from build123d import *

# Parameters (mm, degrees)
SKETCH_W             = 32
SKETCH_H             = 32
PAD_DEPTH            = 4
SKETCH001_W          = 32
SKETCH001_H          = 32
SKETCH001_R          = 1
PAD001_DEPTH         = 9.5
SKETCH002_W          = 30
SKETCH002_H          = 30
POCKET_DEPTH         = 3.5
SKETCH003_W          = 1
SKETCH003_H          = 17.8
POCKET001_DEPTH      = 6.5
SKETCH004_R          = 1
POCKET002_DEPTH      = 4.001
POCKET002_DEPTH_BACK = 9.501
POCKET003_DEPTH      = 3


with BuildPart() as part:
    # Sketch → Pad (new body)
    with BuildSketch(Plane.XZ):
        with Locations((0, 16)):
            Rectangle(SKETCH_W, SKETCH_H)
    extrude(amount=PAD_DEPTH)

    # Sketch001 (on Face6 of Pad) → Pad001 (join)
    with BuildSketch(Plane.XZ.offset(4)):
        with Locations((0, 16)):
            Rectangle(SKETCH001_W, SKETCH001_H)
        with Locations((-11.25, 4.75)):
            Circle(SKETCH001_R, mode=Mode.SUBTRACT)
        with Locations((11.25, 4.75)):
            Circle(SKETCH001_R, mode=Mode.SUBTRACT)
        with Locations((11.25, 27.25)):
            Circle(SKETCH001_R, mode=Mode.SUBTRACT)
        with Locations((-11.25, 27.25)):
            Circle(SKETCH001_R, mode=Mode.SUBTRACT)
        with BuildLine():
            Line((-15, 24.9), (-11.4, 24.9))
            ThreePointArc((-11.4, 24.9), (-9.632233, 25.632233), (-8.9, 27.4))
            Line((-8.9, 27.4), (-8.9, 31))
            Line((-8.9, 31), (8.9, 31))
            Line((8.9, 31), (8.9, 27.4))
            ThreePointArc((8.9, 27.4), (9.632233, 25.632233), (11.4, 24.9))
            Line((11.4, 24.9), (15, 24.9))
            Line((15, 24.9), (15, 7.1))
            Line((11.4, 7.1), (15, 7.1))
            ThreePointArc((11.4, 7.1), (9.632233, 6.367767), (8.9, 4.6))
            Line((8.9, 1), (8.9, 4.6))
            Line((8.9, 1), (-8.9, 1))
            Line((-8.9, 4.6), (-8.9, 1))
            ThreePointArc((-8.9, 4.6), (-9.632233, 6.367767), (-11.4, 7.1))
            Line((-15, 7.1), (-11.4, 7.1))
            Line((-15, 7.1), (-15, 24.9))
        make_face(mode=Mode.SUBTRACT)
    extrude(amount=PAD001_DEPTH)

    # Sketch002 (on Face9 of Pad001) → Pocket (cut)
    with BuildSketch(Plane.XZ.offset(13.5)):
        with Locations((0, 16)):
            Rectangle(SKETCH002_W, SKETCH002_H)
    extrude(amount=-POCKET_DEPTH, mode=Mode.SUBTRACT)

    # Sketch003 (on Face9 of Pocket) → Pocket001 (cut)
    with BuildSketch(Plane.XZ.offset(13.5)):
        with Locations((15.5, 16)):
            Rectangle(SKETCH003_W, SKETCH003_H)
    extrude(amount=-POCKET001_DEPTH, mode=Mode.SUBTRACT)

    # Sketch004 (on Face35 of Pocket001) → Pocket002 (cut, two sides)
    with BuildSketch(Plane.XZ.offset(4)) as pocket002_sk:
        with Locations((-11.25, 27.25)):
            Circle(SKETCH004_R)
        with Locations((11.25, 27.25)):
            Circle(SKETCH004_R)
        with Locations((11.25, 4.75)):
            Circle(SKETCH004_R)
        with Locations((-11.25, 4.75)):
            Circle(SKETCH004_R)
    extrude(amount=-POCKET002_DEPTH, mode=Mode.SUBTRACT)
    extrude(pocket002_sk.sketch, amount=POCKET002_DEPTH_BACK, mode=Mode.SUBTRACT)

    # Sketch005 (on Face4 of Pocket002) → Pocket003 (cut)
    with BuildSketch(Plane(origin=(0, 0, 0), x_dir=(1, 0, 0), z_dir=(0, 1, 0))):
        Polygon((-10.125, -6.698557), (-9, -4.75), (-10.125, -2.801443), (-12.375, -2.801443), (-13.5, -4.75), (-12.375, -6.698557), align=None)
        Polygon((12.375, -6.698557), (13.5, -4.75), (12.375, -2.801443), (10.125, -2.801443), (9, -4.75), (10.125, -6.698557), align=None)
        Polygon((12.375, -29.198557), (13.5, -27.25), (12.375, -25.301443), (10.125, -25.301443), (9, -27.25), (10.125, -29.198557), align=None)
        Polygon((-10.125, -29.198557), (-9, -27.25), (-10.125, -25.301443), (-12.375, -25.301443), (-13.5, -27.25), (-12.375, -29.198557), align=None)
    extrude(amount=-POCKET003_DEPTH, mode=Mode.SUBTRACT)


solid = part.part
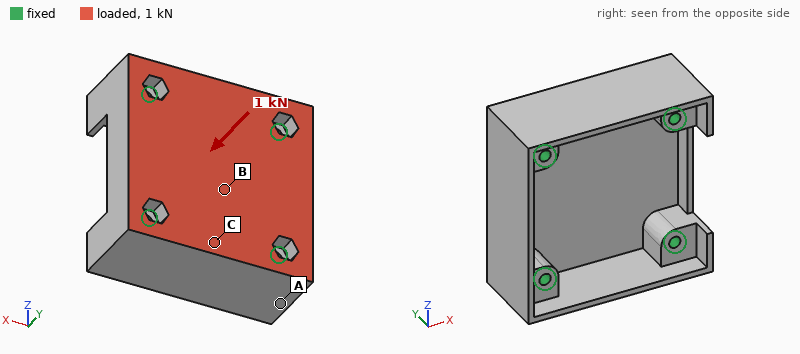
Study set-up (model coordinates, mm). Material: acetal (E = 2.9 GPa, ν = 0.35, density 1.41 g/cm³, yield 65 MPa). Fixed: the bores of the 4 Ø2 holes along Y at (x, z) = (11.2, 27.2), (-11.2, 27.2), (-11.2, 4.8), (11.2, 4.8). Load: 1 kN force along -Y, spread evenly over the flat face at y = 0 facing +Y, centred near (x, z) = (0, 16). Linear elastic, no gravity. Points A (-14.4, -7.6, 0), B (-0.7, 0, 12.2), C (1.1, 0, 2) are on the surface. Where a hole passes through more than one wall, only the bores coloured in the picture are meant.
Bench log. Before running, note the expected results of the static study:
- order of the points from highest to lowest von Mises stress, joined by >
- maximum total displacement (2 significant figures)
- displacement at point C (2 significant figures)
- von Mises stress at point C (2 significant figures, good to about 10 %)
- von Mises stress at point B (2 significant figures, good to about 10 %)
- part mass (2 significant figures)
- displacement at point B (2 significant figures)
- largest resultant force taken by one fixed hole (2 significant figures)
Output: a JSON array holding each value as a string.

["B > C > A", "0.14 mm", "0.049 mm", "6.9 MPa", "11 MPa", "8.1 g", "0.13 mm", "290 N"]
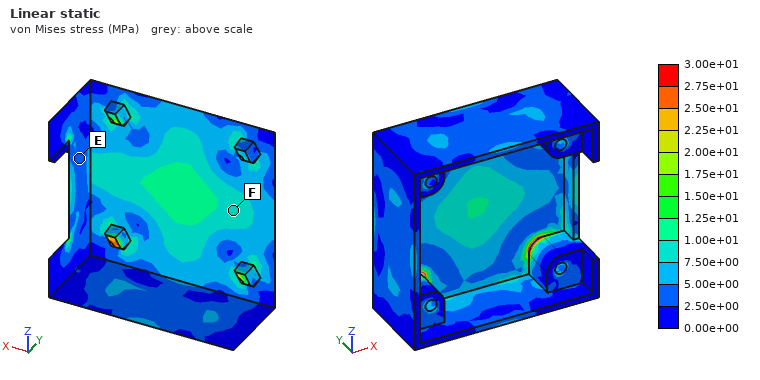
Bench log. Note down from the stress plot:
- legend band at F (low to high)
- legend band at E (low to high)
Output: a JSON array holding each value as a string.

["7.50e+00 to 1.00e+01 MPa", "2.50e+00 to 5.00e+00 MPa"]
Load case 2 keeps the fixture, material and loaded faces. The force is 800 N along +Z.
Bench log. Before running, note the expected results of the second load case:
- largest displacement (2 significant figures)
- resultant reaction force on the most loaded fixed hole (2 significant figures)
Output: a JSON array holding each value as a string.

["42 µm", "210 N"]
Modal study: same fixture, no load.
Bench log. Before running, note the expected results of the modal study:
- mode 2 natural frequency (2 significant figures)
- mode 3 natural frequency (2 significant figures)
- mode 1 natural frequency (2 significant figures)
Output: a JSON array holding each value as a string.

["4800 Hz", "4800 Hz", "4800 Hz"]
